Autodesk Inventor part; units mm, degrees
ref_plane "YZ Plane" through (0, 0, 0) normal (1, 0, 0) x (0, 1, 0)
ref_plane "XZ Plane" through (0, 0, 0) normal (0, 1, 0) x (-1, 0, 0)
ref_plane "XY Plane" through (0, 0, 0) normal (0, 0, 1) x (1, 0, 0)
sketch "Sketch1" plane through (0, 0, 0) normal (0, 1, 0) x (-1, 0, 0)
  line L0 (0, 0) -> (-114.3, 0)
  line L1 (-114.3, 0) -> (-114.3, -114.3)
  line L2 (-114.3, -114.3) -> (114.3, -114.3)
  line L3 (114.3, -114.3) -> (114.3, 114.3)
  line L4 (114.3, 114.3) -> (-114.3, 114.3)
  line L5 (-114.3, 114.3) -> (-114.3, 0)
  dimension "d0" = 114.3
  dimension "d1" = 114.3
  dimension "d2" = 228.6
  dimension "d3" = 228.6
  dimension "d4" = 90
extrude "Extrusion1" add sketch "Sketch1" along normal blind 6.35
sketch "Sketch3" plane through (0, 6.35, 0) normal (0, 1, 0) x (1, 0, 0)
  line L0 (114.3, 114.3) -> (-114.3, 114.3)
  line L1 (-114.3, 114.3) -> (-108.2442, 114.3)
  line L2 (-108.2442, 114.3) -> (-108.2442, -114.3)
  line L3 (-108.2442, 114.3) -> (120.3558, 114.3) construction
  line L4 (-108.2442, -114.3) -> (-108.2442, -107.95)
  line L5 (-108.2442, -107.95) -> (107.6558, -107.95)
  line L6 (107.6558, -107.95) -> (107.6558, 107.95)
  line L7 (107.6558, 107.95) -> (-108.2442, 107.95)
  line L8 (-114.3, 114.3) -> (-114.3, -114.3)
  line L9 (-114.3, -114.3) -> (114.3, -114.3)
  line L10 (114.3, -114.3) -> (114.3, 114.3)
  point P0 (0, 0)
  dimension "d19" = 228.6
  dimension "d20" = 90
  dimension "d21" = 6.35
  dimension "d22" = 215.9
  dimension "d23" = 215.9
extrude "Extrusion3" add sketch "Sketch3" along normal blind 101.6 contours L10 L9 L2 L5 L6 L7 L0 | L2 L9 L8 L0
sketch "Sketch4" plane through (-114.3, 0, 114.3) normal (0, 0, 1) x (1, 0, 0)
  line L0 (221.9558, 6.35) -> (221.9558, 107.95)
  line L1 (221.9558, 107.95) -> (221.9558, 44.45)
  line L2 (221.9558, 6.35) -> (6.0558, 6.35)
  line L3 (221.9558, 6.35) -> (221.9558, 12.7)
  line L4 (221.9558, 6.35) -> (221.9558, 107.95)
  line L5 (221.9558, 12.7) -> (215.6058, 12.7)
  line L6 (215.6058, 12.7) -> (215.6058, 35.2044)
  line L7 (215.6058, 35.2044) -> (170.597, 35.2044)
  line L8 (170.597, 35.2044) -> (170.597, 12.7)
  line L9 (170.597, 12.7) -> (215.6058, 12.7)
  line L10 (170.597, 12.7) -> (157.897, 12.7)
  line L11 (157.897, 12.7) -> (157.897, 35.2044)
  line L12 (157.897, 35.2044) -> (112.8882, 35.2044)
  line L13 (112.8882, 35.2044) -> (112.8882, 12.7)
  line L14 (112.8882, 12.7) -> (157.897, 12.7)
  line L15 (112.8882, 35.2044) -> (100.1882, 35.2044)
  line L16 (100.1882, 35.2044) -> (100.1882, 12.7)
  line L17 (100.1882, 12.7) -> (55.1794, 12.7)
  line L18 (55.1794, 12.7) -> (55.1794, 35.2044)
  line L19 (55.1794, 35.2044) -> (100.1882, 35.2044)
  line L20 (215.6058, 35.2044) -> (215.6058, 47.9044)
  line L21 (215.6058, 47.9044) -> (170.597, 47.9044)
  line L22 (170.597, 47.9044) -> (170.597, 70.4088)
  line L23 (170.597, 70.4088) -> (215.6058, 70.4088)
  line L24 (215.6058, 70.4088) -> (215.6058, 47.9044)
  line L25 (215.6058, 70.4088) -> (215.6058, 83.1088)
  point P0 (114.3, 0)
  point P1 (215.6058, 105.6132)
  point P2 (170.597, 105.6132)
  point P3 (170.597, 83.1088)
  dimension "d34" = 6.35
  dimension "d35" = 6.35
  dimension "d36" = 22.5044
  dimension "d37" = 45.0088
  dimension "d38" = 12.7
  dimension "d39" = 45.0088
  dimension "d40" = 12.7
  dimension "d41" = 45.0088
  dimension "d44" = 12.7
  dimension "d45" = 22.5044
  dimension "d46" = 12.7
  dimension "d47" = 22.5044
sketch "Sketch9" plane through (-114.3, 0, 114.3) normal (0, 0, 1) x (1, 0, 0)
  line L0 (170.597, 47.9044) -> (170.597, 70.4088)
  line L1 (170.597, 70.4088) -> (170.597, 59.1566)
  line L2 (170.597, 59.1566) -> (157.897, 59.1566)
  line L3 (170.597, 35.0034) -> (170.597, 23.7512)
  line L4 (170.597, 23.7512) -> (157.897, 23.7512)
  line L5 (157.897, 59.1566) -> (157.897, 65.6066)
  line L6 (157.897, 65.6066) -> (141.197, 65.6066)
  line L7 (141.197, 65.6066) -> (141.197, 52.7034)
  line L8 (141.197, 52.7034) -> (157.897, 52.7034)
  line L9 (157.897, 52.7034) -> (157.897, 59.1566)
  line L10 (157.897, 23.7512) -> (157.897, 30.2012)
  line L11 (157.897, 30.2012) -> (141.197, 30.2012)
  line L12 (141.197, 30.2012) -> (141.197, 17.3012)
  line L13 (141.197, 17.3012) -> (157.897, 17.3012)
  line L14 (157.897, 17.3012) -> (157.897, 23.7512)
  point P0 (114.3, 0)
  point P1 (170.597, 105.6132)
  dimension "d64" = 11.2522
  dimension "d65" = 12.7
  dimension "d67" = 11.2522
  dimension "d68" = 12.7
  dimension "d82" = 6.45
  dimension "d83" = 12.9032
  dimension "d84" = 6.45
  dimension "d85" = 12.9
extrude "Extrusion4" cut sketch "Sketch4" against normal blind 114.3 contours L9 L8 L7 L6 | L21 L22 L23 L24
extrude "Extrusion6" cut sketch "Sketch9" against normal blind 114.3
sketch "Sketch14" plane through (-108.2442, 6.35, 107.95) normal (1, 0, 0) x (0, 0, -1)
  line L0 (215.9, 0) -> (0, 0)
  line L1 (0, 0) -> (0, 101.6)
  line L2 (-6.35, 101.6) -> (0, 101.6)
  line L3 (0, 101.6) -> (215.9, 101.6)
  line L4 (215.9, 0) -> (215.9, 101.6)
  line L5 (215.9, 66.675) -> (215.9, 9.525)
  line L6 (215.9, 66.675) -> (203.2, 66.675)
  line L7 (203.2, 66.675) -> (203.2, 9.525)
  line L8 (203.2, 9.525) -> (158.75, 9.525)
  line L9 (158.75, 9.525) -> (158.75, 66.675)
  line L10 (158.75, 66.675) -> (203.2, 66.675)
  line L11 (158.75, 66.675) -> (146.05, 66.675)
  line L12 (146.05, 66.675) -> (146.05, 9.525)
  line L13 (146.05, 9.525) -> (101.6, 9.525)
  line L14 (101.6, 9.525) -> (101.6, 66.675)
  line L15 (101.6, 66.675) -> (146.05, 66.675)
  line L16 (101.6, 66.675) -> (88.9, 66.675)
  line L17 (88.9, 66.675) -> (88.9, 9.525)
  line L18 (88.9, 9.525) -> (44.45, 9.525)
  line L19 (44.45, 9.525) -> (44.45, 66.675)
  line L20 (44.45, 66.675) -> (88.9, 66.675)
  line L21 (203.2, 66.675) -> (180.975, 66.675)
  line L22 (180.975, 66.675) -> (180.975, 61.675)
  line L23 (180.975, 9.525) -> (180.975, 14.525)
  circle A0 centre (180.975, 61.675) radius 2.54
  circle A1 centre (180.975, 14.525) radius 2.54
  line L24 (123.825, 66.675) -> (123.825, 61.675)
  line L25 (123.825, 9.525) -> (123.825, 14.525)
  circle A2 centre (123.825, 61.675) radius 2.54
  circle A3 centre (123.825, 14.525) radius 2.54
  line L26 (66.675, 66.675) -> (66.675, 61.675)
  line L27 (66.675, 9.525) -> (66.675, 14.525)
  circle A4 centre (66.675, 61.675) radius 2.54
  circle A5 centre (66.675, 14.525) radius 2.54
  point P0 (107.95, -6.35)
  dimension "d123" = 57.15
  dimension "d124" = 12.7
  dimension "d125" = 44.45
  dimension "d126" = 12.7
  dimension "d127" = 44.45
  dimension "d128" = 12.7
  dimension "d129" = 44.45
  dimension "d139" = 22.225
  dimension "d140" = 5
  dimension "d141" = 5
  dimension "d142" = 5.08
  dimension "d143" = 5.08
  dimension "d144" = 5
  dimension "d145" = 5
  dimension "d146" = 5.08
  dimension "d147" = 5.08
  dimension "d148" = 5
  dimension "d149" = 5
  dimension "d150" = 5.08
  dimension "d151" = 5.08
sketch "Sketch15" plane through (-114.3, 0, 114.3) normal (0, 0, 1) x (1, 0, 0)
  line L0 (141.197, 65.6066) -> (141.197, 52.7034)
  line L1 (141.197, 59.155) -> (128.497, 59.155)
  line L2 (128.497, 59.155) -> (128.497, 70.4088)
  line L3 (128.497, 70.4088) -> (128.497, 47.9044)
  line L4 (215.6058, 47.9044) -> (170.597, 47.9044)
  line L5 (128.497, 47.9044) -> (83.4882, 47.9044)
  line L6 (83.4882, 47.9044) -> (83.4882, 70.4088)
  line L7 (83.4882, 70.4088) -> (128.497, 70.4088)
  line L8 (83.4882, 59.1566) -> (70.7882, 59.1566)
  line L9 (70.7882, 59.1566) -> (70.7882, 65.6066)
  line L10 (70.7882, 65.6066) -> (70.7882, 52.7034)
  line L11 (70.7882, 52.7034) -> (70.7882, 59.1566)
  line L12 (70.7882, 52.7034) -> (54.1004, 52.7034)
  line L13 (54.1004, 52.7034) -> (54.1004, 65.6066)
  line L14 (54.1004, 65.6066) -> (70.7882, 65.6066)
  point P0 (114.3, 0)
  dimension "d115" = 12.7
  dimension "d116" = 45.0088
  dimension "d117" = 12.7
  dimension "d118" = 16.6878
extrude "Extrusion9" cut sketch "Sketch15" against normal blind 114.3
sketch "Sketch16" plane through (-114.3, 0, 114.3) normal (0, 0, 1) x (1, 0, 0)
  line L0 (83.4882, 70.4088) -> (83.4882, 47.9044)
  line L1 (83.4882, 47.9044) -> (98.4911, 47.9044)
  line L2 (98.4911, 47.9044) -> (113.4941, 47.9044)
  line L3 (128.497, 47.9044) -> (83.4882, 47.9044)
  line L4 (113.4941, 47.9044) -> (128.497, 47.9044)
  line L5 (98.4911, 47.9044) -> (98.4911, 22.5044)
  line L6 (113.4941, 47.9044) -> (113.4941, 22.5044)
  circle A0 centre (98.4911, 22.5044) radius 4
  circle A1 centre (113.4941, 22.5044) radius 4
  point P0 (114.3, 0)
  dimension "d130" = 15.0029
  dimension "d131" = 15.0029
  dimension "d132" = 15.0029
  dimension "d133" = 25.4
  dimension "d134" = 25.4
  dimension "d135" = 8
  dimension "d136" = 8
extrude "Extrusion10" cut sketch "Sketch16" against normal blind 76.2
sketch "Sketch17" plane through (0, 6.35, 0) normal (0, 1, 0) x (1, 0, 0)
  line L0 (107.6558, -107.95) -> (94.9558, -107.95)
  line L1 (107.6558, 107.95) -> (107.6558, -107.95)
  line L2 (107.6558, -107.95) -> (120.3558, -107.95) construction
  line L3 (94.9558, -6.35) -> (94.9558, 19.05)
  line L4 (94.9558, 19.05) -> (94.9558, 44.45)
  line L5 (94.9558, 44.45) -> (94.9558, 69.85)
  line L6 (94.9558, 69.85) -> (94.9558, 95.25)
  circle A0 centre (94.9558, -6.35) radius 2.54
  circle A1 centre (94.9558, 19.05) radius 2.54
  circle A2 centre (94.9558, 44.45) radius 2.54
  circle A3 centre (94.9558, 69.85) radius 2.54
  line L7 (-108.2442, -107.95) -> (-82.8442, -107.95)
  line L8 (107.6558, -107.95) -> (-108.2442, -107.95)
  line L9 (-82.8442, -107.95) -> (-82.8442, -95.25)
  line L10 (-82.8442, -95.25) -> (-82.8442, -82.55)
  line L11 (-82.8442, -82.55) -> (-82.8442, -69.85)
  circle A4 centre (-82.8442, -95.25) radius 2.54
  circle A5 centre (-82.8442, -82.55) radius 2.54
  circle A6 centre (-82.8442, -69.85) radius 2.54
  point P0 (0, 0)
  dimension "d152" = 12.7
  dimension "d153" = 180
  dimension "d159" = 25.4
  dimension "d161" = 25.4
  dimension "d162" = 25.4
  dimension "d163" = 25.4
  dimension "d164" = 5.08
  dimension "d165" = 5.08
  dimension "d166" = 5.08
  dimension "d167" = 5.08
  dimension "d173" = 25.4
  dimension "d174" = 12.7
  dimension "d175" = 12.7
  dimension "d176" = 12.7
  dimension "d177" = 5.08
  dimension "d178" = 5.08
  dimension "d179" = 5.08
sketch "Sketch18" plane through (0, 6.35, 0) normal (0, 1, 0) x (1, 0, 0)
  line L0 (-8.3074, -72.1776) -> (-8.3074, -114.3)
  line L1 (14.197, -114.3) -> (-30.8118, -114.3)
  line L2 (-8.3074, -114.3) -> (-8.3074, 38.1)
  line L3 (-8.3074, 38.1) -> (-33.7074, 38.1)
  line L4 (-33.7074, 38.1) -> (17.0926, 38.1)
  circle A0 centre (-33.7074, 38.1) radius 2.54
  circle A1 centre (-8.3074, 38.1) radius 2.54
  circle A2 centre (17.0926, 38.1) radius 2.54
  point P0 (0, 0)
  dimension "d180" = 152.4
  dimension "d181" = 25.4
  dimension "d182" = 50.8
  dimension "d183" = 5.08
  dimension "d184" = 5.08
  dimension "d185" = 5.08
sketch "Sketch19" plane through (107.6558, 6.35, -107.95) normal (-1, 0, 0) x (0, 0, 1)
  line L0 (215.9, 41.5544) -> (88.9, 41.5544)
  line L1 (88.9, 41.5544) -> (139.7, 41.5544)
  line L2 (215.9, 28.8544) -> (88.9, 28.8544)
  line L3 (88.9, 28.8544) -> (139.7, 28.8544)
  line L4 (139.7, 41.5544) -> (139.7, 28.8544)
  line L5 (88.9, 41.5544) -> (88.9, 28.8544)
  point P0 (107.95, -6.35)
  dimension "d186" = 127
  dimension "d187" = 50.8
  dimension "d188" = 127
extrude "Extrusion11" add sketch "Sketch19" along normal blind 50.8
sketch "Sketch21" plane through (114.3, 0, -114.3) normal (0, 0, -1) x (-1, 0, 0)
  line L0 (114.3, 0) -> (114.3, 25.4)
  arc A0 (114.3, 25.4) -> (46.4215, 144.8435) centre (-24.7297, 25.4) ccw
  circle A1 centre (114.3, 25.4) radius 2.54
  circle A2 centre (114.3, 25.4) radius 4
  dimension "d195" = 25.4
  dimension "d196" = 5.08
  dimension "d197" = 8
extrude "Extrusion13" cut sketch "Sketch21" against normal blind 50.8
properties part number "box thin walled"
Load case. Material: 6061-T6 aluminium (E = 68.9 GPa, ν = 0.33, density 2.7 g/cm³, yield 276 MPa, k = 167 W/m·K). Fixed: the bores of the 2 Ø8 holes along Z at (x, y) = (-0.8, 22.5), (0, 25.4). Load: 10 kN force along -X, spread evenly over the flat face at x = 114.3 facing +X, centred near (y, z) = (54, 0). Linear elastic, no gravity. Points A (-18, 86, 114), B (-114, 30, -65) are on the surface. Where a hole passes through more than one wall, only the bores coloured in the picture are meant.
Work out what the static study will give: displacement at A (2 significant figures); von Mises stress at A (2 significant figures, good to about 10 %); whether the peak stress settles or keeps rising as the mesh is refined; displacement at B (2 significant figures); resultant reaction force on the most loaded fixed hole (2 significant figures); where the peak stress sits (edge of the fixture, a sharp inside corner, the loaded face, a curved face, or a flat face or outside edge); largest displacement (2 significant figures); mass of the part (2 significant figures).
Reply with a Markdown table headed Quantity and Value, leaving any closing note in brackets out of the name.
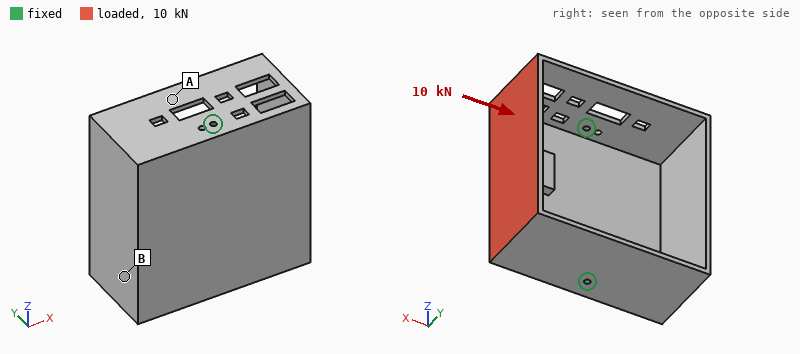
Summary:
| Quantity | Value |
|---|---|
| displacement at A | 0.38 mm |
| von Mises stress at A | 21 MPa |
| whether the peak stress settles or keeps rising as the mesh is refined | keeps rising |
| displacement at B | 0.53 mm |
| resultant reaction force on the most loaded fixed hole | 5.0 kN |
| where the peak stress sits | edge of the fixture |
| largest displacement | 2.2 mm |
| mass of the part | 2.5 kg |
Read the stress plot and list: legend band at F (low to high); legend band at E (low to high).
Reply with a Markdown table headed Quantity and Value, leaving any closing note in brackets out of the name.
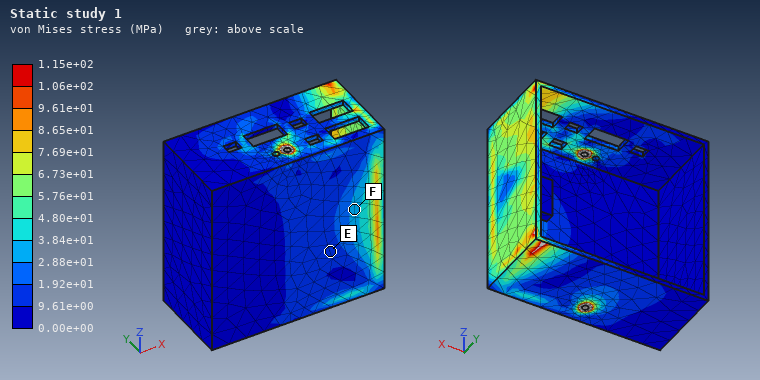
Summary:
| Quantity | Value |
|---|---|
| legend band at F | 2.88e+01 to 3.84e+01 MPa |
| legend band at E | 9.61e+00 to 1.92e+01 MPa |
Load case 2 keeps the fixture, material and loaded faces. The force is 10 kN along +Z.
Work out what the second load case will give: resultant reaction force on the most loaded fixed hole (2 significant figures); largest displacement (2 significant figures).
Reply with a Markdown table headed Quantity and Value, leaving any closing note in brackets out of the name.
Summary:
| Quantity | Value |
|---|---|
| resultant reaction force on the most loaded fixed hole | 7.5 kN |
| largest displacement | 1.4 mm |
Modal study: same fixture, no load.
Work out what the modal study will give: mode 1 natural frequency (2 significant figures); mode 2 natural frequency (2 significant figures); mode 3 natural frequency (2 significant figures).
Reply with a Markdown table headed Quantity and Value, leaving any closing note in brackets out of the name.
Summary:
| Quantity | Value |
|---|---|
| mode 1 natural frequency | 280 Hz |
| mode 2 natural frequency | 390 Hz |
| mode 3 natural frequency | 660 Hz |
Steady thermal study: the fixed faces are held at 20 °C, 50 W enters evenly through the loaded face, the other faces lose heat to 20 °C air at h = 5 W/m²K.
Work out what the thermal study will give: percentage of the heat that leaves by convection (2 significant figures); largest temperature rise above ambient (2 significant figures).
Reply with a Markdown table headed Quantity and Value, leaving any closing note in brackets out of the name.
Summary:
| Quantity | Value |
|---|---|
| percentage of the heat that leaves by convection | 27 % |
| largest temperature rise above ambient | 24 K |
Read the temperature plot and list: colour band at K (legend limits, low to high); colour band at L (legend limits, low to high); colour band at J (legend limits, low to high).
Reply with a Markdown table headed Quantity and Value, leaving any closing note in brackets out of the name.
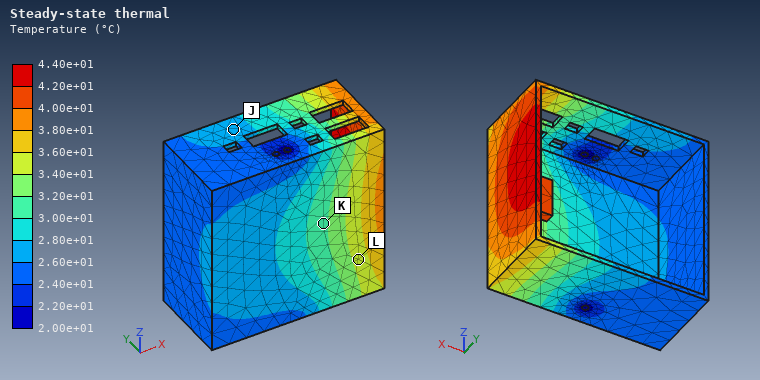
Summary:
| Quantity | Value |
|---|---|
| colour band at K | 3.00e+01 to 3.20e+01 °C |
| colour band at L | 3.40e+01 to 3.60e+01 °C |
| colour band at J | 2.60e+01 to 2.80e+01 °C |
